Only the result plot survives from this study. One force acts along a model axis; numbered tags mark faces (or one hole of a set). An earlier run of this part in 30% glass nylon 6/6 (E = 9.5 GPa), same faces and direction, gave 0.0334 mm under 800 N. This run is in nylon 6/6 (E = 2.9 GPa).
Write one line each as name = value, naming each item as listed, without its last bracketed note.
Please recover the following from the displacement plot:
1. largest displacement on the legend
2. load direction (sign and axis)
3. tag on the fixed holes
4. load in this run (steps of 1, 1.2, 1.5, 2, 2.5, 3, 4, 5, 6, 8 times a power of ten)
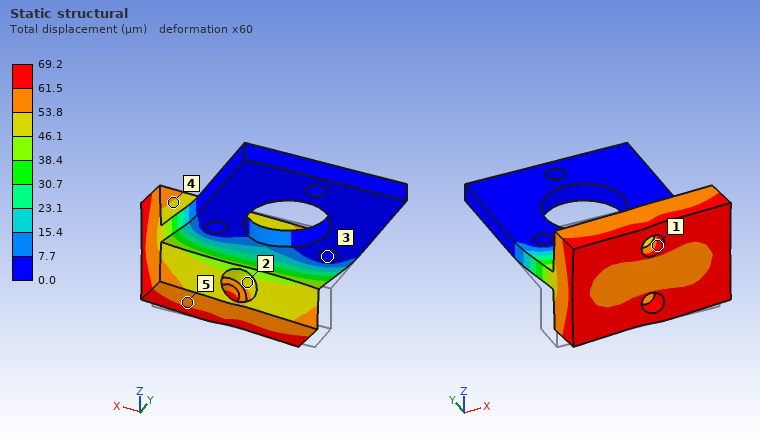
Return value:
largest displacement on the legend = 69.2 µm
load direction = +X
tag on the fixed holes = 3
load in this run = 500 N
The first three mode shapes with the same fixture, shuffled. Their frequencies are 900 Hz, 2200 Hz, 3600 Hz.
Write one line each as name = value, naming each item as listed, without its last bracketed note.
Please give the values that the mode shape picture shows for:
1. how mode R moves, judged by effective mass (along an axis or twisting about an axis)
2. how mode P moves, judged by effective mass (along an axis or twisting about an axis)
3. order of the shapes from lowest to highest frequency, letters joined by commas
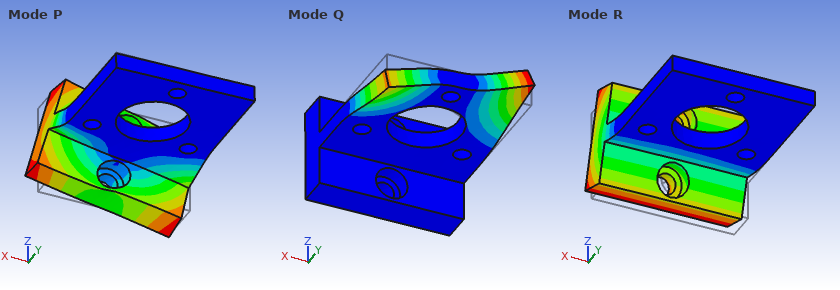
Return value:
how mode R moves, judged by effective mass = along Z
how mode P moves, judged by effective mass = twisting about Y
order of the shapes from lowest to highest frequency, letters joined by commas = R, P, Q
